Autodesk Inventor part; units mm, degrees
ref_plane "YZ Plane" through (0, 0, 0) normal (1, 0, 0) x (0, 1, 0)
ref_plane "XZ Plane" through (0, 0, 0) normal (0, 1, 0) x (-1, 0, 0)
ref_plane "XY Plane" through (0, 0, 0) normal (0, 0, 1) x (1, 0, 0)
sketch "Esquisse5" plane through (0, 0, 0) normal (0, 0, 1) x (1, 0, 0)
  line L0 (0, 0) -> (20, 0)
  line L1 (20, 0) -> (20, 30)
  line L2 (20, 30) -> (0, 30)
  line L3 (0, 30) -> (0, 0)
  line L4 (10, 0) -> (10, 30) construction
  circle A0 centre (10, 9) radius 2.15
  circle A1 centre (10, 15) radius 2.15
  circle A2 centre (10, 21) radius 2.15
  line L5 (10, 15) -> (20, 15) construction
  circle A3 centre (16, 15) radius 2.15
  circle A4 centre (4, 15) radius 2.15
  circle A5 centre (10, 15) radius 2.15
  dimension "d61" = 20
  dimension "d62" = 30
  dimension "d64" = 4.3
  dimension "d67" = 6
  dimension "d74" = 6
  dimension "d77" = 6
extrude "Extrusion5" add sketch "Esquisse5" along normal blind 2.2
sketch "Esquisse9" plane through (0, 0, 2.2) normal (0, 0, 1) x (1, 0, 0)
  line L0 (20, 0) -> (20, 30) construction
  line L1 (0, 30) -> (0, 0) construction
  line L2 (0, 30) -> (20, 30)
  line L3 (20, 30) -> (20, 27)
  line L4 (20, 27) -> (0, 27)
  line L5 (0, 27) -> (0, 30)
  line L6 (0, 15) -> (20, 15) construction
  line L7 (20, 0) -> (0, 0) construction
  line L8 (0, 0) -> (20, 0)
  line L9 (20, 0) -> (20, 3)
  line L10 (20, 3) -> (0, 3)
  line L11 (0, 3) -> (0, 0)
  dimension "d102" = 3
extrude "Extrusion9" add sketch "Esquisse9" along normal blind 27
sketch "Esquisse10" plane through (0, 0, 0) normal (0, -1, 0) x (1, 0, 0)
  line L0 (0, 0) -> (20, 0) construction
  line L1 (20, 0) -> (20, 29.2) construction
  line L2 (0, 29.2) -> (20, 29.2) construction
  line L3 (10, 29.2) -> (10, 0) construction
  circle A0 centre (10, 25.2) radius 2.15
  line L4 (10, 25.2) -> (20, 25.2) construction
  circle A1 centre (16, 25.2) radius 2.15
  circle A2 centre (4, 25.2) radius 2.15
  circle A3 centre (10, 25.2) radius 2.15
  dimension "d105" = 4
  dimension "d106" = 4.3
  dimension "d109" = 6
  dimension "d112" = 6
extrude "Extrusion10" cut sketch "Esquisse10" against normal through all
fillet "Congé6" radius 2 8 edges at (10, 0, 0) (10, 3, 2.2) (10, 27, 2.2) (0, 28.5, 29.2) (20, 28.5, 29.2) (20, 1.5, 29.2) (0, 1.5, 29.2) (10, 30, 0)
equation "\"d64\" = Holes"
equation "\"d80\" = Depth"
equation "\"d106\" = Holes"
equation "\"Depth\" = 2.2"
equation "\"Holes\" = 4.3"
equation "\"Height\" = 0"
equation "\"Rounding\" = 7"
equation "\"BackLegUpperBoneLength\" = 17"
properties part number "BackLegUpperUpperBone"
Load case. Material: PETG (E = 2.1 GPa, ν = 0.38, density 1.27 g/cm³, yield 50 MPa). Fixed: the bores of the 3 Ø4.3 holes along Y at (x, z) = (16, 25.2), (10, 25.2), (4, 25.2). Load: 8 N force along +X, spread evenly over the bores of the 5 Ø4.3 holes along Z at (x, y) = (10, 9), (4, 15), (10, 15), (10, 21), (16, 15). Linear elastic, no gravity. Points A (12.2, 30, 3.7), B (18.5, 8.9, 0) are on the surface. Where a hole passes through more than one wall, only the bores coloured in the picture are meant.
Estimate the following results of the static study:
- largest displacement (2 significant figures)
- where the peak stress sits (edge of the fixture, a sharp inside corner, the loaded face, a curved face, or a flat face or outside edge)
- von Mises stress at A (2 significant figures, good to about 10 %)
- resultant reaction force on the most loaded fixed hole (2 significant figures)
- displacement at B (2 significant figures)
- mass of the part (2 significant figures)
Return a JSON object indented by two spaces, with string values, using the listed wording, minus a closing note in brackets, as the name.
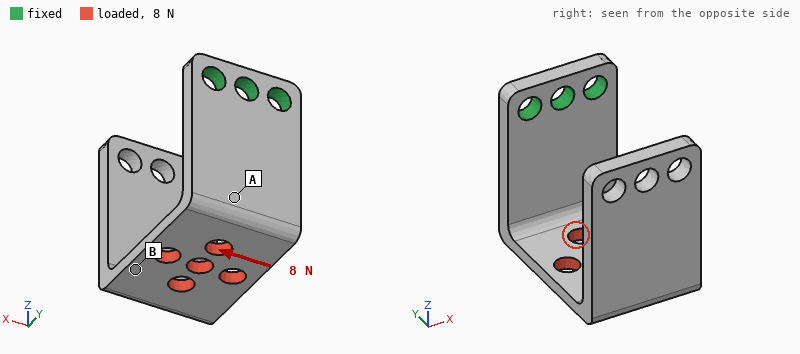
{
  "largest displacement": "0.51 mm",
  "where the peak stress sits": "a flat face or outside edge",
  "von Mises stress at A": "2.2 MPa",
  "resultant reaction force on the most loaded fixed hole": "15 N",
  "displacement at B": "0.30 mm",
  "mass of the part": "5.2 g"
}
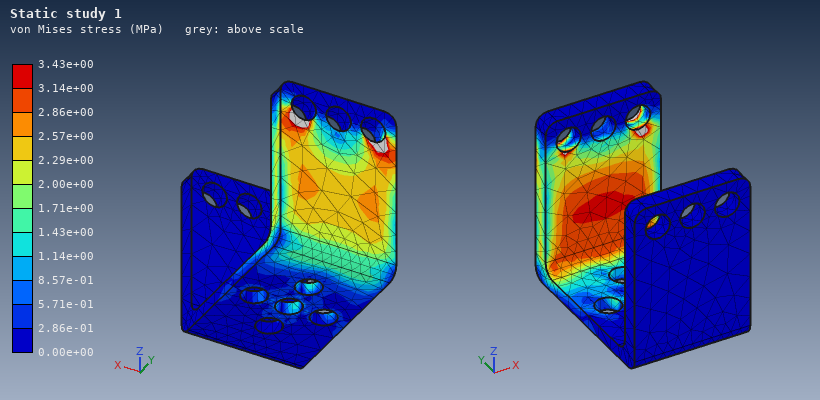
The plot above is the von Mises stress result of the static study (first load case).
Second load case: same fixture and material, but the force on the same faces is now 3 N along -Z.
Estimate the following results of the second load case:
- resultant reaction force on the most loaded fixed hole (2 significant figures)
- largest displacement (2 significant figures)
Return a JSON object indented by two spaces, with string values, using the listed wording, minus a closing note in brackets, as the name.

{
  "resultant reaction force on the most loaded fixed hole": "1.2 N",
  "largest displacement": "0.54 mm"
}
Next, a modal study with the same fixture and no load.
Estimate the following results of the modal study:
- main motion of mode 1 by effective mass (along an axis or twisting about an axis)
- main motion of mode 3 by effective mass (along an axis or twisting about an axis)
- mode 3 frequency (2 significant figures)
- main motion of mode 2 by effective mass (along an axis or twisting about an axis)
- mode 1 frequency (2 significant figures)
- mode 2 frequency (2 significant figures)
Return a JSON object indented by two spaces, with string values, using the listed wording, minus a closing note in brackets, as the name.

{
  "main motion of mode 1 by effective mass": "along Z",
  "main motion of mode 3 by effective mass": "along Y",
  "mode 3 frequency": "360 Hz",
  "main motion of mode 2 by effective mass": "along X",
  "mode 1 frequency": "150 Hz",
  "mode 2 frequency": "230 Hz"
}
